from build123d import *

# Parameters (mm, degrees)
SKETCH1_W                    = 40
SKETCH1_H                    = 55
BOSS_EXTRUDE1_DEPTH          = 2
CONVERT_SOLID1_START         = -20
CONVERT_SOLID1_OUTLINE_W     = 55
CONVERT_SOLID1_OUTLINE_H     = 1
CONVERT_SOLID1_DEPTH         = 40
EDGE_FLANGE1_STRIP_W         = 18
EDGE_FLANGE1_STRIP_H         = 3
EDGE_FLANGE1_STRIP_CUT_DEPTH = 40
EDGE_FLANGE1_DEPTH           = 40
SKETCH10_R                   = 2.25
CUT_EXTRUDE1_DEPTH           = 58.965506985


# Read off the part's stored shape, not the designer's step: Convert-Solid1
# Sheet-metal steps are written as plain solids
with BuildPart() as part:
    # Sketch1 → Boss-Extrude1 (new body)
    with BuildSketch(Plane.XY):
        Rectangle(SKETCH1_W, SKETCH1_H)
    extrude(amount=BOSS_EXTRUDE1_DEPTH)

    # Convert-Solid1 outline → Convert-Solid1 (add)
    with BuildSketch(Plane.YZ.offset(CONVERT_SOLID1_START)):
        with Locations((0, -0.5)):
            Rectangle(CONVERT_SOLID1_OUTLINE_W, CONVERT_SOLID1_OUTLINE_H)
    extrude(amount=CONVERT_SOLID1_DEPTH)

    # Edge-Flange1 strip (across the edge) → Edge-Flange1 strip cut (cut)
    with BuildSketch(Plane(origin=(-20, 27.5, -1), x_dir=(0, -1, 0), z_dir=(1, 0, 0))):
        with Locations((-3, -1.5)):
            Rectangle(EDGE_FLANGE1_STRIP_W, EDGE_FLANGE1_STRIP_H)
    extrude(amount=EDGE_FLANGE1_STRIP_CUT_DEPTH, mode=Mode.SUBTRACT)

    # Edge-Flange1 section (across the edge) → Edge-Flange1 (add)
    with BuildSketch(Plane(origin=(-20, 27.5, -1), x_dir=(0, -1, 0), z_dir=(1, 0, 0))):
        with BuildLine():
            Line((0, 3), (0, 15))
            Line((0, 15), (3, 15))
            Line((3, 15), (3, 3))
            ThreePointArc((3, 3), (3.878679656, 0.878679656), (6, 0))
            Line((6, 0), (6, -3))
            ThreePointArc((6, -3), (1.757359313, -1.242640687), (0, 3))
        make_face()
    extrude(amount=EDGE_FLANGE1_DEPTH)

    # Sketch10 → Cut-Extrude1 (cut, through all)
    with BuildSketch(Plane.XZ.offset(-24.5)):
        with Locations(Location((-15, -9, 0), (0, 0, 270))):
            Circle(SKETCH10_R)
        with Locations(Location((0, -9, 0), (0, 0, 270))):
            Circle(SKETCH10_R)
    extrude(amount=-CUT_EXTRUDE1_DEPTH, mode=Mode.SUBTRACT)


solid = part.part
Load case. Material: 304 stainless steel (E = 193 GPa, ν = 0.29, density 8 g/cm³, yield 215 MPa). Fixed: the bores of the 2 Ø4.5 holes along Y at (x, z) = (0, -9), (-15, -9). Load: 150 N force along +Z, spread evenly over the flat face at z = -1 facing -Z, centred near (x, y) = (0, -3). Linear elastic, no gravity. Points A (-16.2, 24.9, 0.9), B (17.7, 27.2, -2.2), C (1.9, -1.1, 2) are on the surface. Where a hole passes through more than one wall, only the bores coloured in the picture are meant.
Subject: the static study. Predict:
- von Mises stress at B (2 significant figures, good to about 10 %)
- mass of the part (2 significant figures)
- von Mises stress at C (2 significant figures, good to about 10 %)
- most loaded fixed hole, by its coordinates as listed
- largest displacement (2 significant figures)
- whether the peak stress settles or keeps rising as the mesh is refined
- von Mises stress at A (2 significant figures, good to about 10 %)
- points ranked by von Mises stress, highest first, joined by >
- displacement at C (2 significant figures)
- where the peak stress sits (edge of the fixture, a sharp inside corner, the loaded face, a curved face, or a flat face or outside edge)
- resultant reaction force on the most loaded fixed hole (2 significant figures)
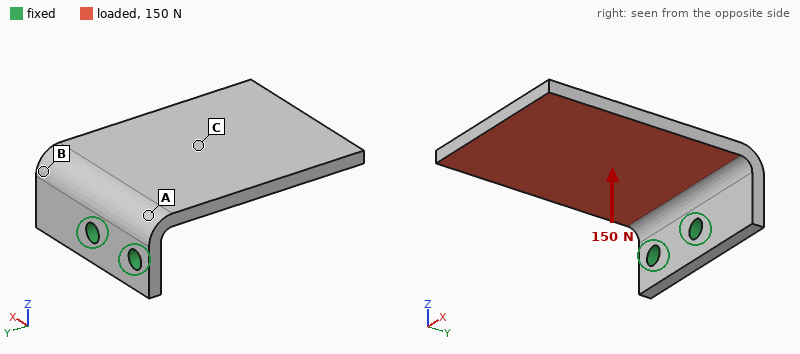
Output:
38 MPa
65 g
17 MPa
(0, -9)
0.28 mm
keeps rising
55 MPa
A > B > C
0.12 mm
edge of the fixture
130 N
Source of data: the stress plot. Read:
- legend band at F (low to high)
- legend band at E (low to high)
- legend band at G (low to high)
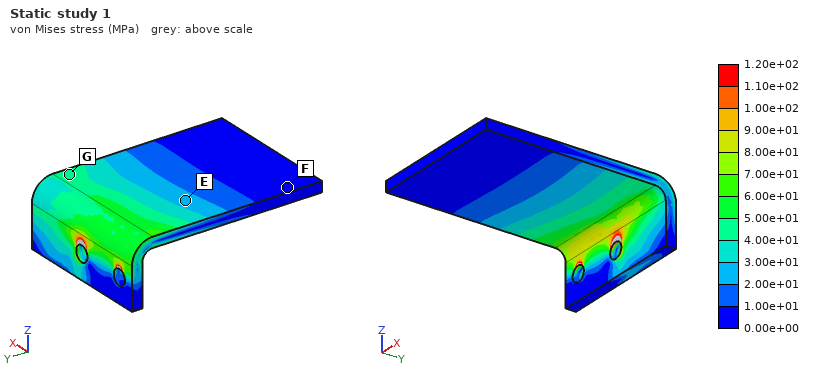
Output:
0.00e+00 to 1.00e+01 MPa
2.00e+01 to 3.00e+01 MPa
4.00e+01 to 5.00e+01 MPa
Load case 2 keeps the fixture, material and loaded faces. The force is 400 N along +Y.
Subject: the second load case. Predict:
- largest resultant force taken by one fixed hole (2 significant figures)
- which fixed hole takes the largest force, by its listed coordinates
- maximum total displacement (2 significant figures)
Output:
350 N
(0, -9)
25 µm
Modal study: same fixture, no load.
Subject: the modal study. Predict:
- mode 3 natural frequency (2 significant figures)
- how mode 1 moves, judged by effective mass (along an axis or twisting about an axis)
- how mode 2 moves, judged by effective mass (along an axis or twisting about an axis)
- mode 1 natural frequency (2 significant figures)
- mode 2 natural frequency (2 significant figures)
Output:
2600 Hz
along Z
along X
660 Hz
1800 Hz
